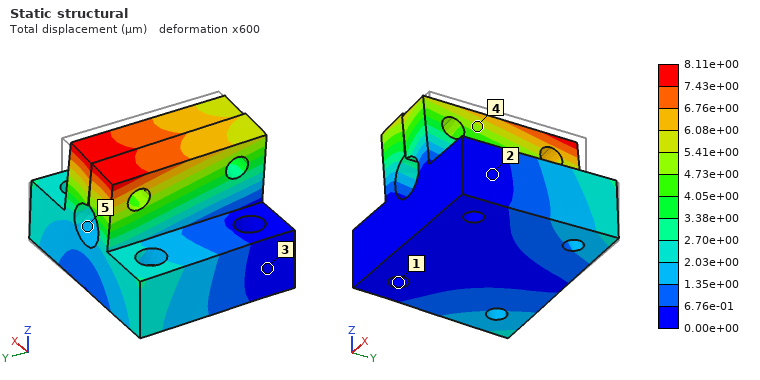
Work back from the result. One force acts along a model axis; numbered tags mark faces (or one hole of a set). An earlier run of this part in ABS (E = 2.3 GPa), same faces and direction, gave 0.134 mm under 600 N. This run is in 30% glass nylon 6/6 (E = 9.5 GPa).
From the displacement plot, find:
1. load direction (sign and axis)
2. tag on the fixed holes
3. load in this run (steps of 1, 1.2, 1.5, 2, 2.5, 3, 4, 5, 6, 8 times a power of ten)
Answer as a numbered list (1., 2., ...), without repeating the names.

1. -X
2. 1
3. 150 N
